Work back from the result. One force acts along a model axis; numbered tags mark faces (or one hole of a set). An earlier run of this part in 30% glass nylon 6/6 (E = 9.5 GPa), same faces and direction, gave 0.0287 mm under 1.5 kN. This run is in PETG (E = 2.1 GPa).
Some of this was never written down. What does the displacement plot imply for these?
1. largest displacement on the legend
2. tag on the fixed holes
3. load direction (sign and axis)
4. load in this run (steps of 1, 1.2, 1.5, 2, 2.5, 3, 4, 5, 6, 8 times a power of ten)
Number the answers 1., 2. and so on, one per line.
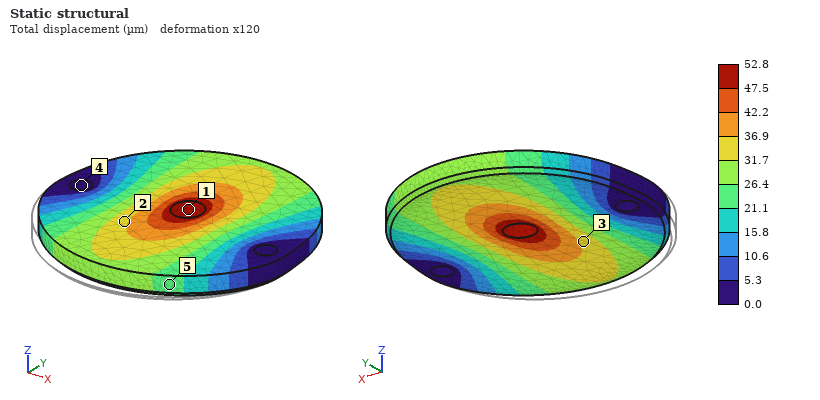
1. 52.8 µm
2. 4
3. +Y
4. 600 N
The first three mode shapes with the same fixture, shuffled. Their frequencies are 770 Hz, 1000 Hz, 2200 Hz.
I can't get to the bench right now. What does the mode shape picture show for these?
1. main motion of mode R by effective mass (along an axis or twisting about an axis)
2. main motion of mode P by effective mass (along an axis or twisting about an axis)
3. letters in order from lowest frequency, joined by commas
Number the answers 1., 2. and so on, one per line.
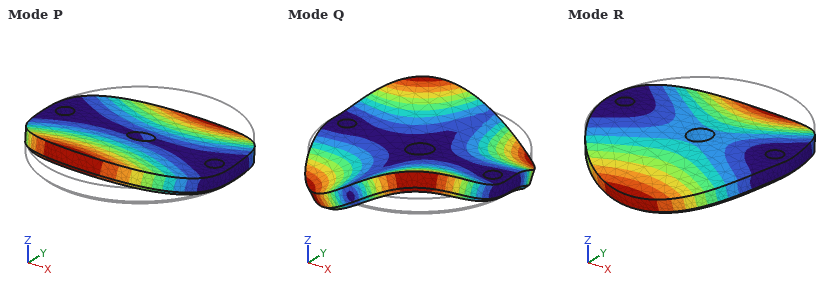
1. along Z
2. twisting about X
3. P, R, Q
